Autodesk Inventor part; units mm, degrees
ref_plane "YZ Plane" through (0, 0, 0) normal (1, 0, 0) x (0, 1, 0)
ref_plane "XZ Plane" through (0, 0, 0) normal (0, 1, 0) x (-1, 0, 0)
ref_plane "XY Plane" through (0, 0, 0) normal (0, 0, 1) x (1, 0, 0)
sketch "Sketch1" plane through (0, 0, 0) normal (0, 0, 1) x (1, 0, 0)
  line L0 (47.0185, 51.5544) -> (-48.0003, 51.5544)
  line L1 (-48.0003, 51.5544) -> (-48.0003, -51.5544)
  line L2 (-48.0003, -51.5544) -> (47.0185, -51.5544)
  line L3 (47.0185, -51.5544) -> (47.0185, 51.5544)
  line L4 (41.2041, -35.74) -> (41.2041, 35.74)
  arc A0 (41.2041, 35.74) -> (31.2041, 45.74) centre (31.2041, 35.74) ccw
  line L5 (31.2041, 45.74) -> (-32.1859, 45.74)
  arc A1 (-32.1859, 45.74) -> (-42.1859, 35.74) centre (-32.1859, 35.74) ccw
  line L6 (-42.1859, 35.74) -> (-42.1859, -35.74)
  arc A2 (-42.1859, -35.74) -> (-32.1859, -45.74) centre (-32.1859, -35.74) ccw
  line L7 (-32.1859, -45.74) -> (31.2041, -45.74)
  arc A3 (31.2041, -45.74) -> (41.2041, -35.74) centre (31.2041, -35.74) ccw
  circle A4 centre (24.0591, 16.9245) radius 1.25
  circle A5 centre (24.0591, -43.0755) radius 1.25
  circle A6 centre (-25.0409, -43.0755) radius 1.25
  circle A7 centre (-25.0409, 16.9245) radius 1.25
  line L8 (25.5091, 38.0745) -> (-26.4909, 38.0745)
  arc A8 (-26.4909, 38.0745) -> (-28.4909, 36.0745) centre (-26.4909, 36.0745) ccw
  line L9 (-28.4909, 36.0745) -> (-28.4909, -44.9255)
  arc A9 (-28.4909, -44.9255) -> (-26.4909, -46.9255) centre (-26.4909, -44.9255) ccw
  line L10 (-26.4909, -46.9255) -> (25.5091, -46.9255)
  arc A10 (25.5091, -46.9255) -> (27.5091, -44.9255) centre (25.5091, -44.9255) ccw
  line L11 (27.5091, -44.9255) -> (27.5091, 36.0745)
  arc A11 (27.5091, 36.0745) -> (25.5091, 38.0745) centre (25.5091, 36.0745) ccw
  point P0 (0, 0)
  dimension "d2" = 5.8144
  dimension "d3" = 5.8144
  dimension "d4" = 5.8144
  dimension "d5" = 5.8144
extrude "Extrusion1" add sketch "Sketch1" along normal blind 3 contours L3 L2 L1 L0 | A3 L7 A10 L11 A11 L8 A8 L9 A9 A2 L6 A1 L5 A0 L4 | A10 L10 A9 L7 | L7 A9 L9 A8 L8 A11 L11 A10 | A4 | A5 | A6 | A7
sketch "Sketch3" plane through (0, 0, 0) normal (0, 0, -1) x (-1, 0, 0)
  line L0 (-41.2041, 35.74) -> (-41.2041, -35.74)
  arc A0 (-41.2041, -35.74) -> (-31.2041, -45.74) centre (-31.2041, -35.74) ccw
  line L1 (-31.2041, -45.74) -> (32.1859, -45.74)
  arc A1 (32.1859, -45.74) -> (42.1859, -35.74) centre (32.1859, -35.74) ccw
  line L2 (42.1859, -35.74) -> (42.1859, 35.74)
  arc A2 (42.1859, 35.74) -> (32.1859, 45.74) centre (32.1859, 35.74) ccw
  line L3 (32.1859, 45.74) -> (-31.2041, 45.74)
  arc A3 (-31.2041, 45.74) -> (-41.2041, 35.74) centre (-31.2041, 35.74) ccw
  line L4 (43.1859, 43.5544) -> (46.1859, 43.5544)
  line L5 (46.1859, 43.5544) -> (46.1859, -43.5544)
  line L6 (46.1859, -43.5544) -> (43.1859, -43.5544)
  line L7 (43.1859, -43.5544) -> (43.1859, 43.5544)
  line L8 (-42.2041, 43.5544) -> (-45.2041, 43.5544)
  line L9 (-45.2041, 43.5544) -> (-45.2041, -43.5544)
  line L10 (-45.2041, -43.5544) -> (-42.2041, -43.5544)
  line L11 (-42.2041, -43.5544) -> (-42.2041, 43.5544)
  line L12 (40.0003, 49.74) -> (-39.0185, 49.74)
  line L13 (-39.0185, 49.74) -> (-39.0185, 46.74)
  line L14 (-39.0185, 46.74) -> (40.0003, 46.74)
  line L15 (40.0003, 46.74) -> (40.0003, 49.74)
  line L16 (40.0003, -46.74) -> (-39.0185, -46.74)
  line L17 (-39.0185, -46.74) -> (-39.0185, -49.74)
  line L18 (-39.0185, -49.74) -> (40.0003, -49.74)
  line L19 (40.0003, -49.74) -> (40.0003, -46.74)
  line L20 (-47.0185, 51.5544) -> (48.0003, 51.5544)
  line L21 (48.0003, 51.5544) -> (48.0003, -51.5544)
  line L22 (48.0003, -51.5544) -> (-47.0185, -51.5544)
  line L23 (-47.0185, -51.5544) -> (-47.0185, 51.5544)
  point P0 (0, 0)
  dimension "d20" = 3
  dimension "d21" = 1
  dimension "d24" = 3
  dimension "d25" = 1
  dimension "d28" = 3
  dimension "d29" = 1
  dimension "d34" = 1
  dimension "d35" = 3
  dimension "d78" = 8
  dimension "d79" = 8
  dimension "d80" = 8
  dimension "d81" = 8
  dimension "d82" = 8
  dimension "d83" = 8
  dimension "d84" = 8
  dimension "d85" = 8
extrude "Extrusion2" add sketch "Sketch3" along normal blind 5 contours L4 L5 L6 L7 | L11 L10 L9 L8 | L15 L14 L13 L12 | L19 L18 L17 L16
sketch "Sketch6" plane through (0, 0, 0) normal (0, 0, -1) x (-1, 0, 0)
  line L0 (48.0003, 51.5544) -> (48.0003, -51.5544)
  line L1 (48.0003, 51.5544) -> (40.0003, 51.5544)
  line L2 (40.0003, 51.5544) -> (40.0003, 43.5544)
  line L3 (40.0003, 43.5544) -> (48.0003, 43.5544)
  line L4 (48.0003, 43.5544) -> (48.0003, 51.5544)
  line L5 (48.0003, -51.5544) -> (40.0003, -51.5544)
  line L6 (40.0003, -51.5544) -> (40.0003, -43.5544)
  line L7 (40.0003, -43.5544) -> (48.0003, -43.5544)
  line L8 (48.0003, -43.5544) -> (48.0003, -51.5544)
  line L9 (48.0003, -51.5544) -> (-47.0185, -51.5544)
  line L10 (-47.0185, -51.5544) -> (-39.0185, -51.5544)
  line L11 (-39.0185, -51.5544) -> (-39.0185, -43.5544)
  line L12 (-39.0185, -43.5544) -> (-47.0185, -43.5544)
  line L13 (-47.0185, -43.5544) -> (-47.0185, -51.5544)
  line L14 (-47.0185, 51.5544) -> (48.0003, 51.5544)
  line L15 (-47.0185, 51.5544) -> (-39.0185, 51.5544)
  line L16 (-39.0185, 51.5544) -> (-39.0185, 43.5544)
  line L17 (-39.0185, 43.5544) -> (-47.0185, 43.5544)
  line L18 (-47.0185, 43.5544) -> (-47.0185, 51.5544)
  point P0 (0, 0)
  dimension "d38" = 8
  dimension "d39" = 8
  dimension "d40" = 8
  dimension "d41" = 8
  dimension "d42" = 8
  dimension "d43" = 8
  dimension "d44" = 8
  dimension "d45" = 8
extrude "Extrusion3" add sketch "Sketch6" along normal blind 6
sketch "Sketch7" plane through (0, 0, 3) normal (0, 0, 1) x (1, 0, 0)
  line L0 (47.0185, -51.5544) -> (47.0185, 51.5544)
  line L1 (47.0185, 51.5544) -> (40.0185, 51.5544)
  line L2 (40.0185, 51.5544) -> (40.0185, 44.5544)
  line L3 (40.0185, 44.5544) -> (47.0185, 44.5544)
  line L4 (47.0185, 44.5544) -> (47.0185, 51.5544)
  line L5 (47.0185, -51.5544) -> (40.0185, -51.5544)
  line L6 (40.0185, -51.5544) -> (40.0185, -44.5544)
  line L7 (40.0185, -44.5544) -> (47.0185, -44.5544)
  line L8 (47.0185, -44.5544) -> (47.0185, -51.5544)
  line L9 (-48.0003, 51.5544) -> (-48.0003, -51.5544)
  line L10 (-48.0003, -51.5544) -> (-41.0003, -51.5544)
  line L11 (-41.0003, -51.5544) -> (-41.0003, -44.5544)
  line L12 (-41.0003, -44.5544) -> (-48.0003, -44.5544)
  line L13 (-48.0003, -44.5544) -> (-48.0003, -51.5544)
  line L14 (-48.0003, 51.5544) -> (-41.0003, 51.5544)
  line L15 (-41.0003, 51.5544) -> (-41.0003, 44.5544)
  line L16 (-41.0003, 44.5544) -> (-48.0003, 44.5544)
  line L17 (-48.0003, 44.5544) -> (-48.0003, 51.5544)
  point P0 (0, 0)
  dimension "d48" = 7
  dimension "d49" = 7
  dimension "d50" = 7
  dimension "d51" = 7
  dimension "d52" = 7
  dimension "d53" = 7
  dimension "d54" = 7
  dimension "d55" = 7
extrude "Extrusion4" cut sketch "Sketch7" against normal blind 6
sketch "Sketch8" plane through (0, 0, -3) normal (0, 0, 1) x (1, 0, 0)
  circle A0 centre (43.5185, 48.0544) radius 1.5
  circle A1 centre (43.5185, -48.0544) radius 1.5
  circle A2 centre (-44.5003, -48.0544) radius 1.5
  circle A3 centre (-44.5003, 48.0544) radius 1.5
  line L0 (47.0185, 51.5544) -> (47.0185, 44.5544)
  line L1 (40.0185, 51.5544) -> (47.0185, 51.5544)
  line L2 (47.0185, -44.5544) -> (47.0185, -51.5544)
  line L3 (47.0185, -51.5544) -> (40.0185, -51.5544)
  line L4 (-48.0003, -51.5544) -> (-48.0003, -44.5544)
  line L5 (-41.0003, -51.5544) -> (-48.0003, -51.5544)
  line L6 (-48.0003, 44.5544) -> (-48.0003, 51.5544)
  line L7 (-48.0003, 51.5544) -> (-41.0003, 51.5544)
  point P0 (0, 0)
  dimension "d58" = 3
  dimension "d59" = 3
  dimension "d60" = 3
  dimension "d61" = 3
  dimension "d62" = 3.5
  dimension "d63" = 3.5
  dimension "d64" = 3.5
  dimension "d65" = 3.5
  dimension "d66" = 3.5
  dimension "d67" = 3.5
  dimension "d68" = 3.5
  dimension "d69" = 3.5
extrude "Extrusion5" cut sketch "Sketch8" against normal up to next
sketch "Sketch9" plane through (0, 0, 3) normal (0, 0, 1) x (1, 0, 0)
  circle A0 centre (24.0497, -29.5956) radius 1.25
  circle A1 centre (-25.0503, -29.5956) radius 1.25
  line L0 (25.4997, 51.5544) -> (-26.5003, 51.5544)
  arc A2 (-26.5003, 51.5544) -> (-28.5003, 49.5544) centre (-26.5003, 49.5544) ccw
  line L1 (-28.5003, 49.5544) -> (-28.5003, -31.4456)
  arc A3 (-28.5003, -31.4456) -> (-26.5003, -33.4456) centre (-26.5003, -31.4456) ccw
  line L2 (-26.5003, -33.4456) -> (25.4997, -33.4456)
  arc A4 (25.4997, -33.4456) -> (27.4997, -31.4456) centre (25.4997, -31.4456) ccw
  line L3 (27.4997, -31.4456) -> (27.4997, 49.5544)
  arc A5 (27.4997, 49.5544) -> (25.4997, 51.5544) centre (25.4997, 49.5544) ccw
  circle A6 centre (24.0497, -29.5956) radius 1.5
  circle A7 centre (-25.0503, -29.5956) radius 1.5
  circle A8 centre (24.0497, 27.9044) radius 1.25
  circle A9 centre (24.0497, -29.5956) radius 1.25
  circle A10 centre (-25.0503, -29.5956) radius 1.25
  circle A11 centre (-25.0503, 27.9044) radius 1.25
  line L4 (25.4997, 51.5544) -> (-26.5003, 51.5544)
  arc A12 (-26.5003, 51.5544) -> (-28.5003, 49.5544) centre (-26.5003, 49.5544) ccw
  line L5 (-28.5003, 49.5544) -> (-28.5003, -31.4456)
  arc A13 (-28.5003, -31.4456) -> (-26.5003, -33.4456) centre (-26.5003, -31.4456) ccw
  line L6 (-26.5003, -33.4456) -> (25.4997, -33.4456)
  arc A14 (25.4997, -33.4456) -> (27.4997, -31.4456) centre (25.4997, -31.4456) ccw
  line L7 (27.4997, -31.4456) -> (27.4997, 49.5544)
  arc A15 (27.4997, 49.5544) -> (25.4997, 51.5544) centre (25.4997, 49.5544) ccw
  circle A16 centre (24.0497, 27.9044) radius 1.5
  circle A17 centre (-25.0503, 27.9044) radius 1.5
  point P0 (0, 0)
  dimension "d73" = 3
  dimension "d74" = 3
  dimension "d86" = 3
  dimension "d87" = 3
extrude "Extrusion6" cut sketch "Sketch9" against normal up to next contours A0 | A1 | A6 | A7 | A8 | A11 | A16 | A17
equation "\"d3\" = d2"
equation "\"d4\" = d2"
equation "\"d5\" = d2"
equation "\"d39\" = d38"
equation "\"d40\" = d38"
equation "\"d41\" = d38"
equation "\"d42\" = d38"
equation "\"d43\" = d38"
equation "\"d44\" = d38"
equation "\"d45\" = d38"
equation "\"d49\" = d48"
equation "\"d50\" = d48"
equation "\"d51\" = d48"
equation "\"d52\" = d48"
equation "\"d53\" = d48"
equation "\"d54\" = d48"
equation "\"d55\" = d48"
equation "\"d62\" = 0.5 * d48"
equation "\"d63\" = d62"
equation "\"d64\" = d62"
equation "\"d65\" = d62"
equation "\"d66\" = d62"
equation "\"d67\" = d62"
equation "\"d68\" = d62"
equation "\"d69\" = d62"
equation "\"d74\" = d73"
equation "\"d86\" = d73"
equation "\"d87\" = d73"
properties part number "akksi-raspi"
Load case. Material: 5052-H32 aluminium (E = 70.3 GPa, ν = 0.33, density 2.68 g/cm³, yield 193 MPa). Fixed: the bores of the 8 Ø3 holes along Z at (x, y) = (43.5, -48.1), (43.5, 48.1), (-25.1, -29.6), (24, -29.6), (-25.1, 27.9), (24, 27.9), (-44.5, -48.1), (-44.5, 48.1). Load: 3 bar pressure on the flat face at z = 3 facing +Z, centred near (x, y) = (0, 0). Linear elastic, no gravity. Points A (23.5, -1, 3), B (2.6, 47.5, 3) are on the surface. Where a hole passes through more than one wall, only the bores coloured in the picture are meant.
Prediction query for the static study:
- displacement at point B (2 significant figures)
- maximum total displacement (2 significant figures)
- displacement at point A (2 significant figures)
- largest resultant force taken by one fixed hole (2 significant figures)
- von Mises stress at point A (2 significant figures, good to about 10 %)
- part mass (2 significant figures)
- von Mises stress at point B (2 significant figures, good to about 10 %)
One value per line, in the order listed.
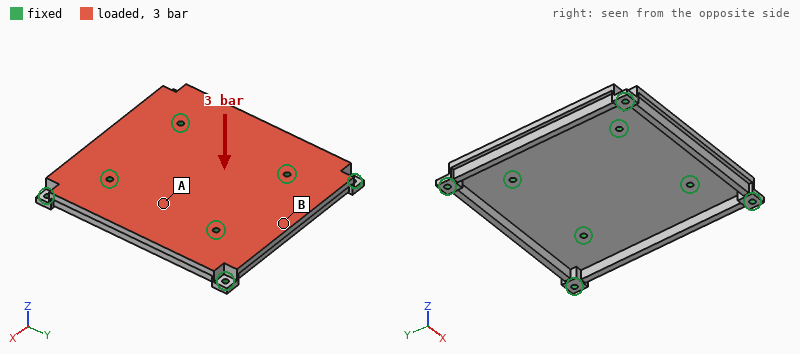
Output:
24 µm
89 µm
62 µm
570 N
25 MPa
93 g
12 MPa
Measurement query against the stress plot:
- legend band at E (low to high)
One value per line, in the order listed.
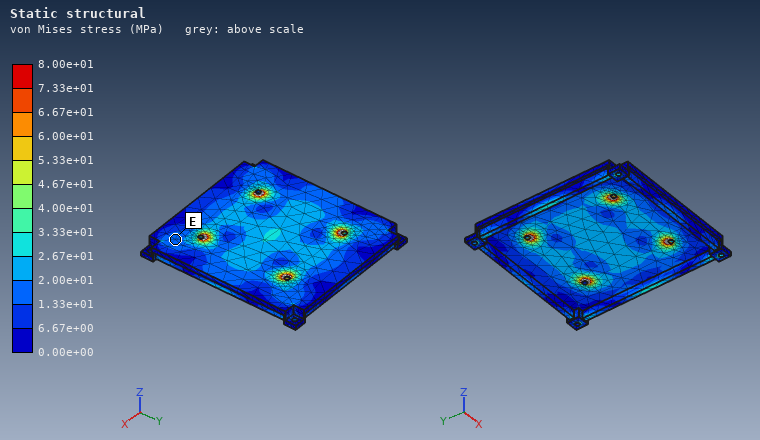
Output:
1.33e+01 to 2.00e+01 MPa
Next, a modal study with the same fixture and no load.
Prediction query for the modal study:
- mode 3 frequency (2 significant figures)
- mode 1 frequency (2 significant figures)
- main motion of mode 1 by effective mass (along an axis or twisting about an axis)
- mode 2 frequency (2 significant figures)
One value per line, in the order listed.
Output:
4500 Hz
4000 Hz
along Z
4500 Hz
